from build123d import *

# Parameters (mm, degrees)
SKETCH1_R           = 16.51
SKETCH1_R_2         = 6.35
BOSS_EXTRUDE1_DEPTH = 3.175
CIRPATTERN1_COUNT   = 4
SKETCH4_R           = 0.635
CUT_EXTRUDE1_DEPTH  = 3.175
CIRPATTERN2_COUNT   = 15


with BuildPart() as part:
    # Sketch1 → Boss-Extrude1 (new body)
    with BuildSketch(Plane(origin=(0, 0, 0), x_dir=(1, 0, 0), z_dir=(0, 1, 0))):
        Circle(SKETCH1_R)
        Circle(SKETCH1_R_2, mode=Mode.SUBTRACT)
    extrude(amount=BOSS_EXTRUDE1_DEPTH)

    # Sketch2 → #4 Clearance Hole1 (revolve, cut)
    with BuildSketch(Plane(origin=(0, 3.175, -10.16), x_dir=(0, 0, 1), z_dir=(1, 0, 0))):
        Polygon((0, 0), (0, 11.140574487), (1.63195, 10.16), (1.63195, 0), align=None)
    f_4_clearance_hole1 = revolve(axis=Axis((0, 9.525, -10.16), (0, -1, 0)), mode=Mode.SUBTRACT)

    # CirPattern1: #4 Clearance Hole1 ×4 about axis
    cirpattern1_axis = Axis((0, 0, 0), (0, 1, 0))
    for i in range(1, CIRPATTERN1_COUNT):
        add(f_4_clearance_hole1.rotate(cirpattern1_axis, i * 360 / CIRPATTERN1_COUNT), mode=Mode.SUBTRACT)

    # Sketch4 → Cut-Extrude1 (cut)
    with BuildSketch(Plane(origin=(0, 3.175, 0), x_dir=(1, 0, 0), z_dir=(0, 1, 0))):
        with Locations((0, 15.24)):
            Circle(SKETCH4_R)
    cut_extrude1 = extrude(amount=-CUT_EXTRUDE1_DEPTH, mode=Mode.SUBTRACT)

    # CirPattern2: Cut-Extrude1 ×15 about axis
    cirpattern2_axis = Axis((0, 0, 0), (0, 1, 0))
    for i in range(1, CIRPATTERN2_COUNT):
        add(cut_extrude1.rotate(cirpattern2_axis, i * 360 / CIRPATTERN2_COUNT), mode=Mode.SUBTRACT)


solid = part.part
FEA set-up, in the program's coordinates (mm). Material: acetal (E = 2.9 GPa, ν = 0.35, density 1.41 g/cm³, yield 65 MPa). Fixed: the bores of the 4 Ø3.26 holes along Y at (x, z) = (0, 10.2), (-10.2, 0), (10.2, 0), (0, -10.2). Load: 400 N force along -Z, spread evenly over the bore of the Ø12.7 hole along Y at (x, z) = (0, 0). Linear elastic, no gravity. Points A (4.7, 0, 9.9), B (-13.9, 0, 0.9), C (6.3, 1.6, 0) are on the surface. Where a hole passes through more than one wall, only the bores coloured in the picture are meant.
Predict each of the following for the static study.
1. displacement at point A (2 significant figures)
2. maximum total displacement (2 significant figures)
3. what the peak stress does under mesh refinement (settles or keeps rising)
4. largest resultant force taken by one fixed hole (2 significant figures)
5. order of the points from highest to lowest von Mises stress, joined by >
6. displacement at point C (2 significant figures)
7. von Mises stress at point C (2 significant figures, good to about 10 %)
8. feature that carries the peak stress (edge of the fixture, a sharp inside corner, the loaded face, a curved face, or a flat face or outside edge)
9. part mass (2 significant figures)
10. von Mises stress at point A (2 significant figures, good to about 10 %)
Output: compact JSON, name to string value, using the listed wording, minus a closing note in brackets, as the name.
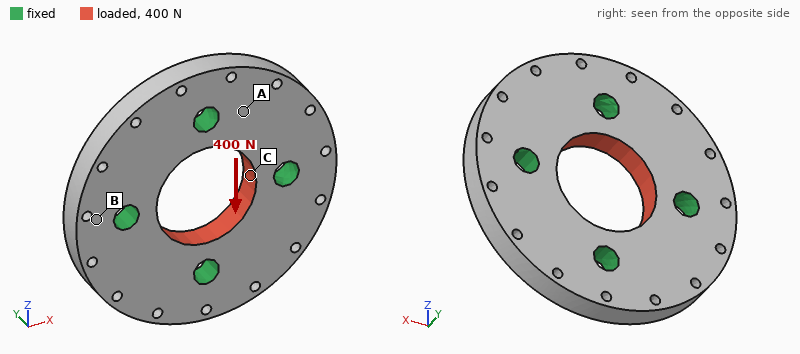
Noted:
{"displacement at point A": "4.5 µm", "maximum total displacement": "9.6 µm", "what the peak stress does under mesh refinement": "keeps rising", "largest resultant force taken by one fixed hole": "100 N", "order of the points from highest to lowest von Mises stress, joined by >": "C > A > B", "displacement at point C": "8.5 µm", "von Mises stress at point C": "5.6 MPa", "feature that carries the peak stress": "edge of the fixture", "part mass": "3.0 g", "von Mises stress at point A": "1.9 MPa"}
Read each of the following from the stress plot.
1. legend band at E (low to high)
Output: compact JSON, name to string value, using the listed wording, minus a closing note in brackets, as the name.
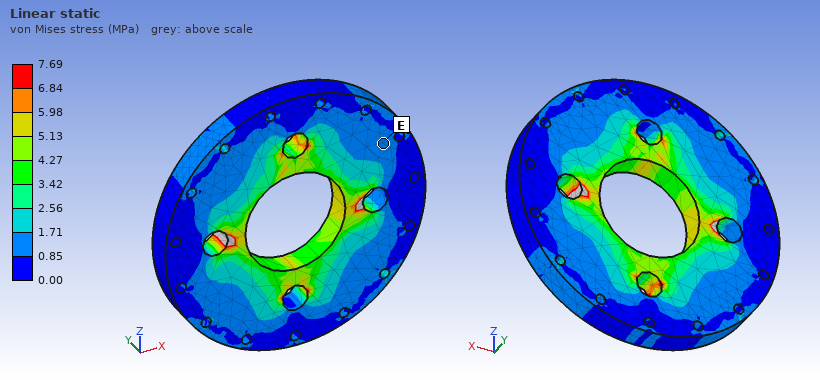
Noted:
{"legend band at E": "0.85 to 1.71 MPa"}
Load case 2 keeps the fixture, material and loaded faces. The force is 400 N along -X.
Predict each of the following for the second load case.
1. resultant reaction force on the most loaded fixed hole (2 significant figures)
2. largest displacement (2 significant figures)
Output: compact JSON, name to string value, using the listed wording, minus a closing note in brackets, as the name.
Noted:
{"resultant reaction force on the most loaded fixed hole": "100 N", "largest displacement": "9.6 µm"}
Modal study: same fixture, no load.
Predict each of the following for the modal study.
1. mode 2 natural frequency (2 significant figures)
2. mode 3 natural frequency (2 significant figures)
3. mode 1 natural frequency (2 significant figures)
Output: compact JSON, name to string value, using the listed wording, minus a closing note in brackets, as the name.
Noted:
{"mode 2 natural frequency": "9700 Hz", "mode 3 natural frequency": "9700 Hz", "mode 1 natural frequency": "9200 Hz"}
